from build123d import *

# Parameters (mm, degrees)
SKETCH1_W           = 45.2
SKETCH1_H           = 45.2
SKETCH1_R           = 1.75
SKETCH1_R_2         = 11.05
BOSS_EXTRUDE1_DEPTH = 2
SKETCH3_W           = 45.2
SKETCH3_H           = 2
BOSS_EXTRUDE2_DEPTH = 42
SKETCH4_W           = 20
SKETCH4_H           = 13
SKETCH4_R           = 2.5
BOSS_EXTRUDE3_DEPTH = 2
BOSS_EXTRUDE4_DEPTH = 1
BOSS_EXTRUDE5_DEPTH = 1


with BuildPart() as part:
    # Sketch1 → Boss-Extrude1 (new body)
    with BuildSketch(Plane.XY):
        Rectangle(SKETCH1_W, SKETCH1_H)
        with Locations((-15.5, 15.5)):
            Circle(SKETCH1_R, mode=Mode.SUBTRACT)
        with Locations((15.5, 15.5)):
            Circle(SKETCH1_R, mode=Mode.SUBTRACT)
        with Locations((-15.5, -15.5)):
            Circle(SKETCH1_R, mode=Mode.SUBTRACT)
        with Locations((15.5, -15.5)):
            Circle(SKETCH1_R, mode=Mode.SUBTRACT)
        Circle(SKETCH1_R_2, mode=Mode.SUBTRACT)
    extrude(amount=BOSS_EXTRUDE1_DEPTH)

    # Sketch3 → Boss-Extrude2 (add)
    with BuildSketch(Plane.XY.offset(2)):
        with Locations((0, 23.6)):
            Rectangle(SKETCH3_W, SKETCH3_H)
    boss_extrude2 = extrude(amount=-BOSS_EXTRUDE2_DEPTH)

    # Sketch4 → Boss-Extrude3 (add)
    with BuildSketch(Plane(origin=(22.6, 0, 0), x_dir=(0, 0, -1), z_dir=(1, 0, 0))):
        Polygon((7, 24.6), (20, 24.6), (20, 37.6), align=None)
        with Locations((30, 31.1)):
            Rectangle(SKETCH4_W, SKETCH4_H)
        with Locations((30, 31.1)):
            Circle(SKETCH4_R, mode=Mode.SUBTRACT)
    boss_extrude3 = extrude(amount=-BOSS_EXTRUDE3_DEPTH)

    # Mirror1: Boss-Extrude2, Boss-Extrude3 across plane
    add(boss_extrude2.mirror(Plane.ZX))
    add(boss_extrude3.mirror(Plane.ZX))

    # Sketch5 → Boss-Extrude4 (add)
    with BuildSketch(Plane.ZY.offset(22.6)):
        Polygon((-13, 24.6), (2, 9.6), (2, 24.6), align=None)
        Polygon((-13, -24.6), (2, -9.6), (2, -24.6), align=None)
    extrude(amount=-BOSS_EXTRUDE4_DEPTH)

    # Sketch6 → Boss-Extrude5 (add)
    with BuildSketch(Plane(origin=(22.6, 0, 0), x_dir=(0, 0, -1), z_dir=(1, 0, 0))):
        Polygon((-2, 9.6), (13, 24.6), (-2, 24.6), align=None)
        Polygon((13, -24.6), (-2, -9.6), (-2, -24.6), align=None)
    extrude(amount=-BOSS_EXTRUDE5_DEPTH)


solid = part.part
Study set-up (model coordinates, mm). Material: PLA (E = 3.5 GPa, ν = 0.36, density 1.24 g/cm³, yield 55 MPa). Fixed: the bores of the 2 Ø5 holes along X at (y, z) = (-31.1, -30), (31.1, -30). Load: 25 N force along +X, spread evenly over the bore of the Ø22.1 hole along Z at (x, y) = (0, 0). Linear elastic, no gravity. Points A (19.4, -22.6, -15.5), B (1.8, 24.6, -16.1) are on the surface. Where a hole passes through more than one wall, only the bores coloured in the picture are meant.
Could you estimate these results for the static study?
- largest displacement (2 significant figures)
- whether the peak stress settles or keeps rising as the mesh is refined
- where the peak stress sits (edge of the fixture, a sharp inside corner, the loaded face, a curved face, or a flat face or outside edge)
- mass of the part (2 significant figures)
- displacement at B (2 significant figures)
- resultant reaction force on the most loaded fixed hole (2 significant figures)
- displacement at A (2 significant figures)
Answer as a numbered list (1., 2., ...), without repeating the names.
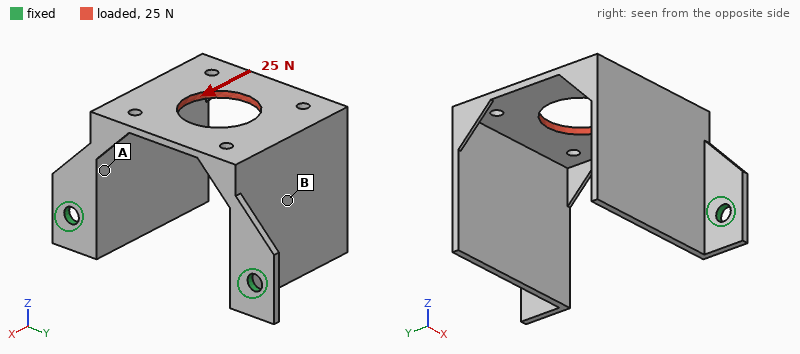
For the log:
1. 1.1 mm
2. keeps rising
3. edge of the fixture
4. 15 g
5. 0.48 mm
6. 13 N
7. 0.30 mm
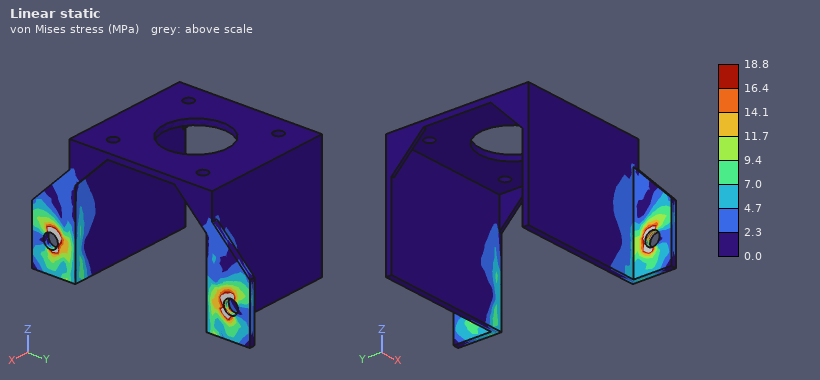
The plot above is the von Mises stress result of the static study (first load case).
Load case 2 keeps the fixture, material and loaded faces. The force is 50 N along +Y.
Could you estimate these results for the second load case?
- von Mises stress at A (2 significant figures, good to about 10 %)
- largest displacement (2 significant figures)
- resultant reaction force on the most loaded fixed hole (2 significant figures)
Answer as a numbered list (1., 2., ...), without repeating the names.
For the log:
1. 6.1 MPa
2. 1.2 mm
3. 32 N
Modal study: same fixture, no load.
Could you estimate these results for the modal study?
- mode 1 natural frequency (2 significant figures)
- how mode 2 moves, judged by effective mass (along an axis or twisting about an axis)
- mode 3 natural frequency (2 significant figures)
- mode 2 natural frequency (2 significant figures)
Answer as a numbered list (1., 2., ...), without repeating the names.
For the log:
1. 250 Hz
2. along Y
3. 460 Hz
4. 280 Hz
